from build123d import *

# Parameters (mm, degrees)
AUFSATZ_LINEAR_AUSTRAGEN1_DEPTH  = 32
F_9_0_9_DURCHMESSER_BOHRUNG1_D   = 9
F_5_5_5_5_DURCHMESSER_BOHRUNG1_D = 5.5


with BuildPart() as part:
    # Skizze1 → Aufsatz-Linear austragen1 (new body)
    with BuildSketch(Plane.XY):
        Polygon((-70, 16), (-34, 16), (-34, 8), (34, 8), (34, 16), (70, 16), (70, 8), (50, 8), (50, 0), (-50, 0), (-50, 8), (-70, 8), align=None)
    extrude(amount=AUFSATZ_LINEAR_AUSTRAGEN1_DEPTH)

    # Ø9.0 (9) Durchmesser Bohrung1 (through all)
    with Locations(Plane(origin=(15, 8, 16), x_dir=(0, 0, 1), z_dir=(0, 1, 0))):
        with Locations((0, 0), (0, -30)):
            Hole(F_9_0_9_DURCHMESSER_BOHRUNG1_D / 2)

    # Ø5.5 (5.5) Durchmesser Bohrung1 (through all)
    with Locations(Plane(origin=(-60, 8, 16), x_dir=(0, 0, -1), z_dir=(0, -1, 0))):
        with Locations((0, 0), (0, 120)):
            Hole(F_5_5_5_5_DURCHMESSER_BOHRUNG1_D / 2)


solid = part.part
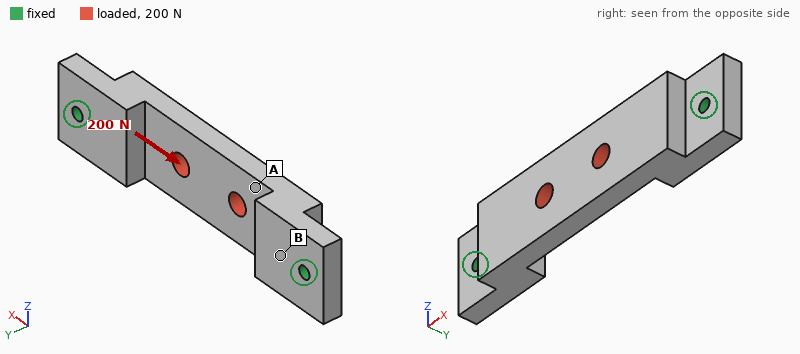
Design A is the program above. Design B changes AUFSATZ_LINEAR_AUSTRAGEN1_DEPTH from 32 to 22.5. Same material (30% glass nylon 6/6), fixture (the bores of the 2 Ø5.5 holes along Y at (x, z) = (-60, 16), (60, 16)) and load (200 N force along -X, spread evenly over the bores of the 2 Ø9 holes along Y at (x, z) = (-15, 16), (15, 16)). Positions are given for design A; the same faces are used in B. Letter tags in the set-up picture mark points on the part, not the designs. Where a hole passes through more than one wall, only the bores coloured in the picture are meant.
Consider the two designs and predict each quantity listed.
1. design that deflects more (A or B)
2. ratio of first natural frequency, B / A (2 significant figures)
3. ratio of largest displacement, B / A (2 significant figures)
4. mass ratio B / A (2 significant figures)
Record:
B
0.89
1.6
0.69
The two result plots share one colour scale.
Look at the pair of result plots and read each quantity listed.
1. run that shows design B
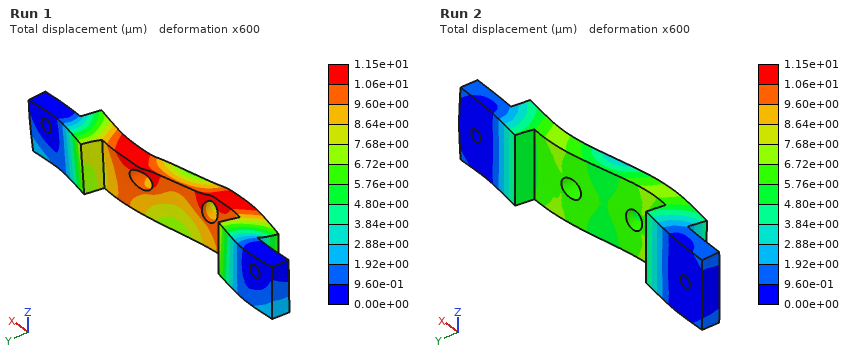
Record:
Run 1
